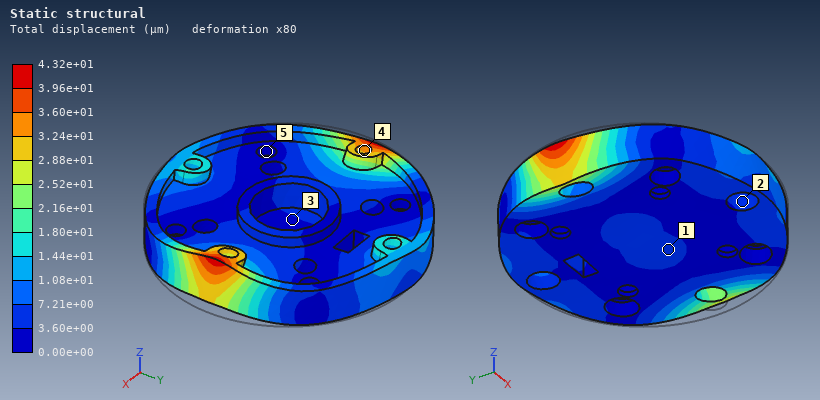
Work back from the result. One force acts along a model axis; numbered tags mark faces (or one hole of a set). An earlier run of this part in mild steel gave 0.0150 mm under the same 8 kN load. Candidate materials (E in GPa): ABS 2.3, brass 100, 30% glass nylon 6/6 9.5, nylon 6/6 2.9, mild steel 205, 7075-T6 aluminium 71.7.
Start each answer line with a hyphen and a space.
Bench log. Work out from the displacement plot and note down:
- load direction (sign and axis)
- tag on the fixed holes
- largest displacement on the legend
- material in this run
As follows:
- -X
- 5
- 4.32e+01 µm
- 7075-T6 aluminium
